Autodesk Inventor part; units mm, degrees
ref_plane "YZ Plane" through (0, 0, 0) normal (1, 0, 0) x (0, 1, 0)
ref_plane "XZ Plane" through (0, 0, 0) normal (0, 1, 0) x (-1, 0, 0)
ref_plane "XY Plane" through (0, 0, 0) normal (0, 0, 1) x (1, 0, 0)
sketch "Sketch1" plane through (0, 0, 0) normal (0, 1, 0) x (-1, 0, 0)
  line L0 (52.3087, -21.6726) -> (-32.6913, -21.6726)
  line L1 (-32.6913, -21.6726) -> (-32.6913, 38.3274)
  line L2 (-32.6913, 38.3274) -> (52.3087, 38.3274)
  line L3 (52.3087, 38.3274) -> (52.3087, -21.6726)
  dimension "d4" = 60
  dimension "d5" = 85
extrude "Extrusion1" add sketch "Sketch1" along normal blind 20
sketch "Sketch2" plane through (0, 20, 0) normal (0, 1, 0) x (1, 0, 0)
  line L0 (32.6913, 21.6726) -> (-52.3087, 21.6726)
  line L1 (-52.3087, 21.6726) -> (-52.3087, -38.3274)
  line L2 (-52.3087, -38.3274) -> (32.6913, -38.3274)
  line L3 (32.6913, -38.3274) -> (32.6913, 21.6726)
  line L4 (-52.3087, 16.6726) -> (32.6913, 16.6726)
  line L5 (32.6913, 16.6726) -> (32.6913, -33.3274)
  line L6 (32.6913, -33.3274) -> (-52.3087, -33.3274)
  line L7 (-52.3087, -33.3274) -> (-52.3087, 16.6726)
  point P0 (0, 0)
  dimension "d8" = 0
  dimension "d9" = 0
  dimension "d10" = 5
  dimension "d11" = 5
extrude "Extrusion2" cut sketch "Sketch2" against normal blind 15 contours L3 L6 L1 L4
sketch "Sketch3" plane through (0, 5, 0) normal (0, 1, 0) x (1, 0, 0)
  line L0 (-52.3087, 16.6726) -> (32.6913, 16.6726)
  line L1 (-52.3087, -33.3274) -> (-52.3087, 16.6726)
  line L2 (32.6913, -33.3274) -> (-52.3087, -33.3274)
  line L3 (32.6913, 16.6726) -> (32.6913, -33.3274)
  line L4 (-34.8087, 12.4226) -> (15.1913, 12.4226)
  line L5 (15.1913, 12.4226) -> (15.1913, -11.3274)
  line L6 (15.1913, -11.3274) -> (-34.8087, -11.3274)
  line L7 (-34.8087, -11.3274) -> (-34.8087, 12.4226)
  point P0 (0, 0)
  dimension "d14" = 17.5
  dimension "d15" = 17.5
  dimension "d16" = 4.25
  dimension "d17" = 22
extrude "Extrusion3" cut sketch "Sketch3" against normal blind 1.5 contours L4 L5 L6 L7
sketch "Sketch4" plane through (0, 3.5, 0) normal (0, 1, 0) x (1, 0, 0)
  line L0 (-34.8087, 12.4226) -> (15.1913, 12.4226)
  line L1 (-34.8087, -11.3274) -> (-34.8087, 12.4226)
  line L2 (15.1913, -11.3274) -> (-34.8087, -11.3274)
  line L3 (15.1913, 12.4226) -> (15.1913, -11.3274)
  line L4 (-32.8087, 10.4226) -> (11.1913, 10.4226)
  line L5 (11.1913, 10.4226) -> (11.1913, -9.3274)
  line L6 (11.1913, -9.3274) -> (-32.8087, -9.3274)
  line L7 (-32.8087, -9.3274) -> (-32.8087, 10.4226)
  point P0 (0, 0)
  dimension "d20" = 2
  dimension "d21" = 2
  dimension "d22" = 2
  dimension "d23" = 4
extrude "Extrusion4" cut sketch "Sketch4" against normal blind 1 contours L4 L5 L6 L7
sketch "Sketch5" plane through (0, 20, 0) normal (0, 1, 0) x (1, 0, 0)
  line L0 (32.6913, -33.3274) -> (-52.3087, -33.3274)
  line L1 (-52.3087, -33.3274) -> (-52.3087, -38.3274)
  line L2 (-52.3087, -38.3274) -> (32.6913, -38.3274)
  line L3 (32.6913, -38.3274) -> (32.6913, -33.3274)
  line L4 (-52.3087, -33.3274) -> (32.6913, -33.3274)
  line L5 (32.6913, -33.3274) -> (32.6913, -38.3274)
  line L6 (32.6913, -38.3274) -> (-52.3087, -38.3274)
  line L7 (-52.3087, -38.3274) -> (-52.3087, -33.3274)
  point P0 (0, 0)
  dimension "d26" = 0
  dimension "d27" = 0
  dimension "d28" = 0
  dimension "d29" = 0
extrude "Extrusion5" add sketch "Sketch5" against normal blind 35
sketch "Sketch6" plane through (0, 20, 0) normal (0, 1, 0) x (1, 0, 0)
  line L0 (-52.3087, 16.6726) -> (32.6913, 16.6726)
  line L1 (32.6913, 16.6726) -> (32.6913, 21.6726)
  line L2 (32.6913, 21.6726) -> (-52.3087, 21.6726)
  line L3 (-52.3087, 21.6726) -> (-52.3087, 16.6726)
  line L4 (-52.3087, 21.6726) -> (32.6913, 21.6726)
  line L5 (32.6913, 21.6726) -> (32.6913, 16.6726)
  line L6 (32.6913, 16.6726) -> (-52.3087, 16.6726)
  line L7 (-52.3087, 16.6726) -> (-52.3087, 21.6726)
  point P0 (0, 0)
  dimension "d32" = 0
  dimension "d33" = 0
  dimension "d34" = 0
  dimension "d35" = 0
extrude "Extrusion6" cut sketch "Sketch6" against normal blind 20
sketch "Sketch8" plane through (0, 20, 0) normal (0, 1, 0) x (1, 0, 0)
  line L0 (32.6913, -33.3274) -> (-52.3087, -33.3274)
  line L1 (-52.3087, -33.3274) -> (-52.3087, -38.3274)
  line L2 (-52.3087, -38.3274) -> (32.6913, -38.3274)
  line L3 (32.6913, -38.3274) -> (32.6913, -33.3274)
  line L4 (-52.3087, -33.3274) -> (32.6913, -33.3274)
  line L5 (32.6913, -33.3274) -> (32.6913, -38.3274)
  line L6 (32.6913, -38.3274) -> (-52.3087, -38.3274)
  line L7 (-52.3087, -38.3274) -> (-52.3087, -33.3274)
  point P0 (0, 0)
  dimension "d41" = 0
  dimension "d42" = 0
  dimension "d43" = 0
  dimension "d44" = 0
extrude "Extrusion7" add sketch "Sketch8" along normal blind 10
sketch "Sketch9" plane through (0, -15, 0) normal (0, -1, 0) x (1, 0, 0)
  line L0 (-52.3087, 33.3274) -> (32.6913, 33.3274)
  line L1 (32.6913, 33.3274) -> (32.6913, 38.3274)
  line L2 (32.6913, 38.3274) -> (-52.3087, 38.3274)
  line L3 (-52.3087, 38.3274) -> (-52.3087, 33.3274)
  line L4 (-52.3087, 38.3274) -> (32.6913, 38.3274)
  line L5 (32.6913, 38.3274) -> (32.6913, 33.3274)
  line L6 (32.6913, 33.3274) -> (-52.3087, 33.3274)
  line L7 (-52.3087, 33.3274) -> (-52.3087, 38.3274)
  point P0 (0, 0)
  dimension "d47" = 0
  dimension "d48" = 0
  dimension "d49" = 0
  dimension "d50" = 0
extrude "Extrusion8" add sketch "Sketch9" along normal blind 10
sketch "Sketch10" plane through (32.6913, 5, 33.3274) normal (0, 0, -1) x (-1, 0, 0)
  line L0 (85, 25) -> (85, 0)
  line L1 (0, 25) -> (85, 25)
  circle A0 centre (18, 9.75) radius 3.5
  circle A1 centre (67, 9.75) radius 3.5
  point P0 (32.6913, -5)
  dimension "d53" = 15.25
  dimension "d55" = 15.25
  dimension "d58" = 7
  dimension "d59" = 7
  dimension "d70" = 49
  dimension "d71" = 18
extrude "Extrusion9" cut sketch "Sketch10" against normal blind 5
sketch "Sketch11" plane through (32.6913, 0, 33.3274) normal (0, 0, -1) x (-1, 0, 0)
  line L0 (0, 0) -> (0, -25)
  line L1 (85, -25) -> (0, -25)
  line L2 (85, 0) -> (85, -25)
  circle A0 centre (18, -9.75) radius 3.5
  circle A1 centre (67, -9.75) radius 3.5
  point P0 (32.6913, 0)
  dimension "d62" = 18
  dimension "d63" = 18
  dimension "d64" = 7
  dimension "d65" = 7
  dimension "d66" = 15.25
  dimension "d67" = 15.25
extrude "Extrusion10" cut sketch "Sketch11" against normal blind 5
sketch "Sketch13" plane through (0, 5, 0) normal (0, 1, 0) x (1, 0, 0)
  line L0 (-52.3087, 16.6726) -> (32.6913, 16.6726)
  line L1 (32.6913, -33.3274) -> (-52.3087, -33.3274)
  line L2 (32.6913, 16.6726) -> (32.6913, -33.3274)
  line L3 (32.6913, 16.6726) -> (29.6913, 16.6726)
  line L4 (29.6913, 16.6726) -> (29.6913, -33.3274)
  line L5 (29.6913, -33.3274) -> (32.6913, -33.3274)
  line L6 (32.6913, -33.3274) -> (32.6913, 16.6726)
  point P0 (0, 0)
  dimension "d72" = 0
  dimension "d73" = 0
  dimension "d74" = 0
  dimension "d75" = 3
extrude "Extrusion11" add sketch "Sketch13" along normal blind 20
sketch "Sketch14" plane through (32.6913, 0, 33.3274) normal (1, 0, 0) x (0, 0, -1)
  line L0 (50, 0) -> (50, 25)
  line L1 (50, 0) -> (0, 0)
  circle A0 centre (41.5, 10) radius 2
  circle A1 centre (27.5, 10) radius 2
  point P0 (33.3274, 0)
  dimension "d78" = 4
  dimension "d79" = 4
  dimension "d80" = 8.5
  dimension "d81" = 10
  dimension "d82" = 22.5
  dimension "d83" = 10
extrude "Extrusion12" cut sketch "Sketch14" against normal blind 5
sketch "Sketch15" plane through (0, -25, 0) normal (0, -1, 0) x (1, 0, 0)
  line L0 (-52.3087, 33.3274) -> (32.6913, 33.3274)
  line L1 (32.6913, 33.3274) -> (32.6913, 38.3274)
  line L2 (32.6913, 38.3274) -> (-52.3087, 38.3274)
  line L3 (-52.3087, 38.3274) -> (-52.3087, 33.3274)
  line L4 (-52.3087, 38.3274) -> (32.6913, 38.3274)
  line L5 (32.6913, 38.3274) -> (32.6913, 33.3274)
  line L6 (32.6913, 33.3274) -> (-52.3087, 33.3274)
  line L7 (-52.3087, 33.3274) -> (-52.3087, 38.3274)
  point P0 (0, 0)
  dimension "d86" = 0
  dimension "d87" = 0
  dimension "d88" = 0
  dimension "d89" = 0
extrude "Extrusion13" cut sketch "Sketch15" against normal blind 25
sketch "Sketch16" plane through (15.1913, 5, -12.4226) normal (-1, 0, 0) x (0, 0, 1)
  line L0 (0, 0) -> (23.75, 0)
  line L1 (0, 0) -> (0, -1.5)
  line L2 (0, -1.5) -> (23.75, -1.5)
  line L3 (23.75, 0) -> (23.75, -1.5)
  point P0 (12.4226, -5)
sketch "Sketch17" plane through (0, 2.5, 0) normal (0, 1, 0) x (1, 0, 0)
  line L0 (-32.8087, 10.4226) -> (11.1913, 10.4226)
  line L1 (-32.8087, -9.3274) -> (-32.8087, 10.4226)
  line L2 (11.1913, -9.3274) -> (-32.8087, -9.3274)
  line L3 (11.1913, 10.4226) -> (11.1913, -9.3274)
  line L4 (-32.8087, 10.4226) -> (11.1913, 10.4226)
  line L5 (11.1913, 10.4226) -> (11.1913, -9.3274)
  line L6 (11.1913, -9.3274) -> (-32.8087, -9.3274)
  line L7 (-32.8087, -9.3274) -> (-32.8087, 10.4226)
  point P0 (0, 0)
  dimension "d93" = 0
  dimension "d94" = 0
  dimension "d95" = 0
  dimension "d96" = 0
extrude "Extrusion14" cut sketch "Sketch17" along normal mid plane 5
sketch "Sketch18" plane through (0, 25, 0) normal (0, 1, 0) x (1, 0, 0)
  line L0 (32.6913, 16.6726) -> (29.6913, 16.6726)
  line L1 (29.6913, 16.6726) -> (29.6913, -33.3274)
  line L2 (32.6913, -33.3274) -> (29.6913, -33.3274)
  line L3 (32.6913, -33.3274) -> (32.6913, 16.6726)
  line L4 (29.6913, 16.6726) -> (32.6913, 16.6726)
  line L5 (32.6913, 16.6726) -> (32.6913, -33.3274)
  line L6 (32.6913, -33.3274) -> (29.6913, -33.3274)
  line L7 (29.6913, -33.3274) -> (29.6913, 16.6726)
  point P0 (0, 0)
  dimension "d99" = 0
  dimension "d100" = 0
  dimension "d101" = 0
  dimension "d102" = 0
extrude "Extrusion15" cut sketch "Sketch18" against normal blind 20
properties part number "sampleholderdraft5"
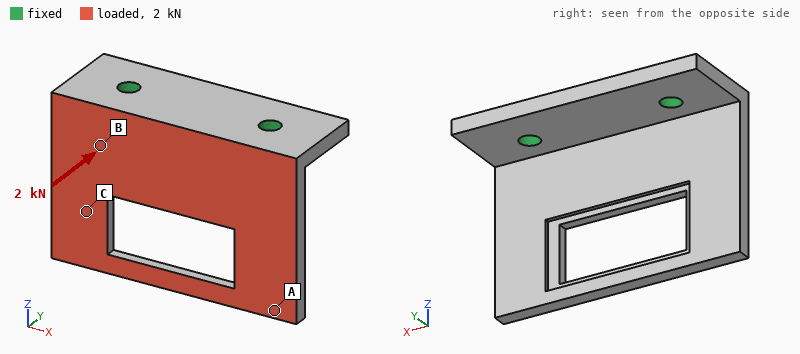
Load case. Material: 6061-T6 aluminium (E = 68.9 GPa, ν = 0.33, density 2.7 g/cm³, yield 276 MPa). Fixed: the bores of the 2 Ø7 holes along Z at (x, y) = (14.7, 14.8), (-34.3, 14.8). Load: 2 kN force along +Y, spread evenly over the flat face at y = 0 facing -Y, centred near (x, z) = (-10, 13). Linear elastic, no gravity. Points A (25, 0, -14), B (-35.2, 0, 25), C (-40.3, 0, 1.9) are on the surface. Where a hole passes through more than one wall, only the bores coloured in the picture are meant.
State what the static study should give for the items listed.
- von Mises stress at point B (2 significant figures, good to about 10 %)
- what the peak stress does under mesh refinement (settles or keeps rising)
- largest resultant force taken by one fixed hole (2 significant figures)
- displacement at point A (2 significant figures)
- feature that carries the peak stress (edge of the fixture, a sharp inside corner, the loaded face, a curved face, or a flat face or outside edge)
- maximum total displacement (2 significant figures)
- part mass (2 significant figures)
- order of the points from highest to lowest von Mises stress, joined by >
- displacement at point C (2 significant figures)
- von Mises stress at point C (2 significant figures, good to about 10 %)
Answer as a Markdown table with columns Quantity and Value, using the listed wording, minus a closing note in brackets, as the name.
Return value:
| Quantity | Value |
|---|---|
| von Mises stress at point B | 77 MPa |
| what the peak stress does under mesh refinement | keeps rising |
| largest resultant force taken by one fixed hole | 1.0 kN |
| displacement at point A | 0.96 mm |
| feature that carries the peak stress | edge of the fixture |
| maximum total displacement | 1.0 mm |
| part mass | 78 g |
| order of the points from highest to lowest von Mises stress, joined by > | B > C > A |
| displacement at point C | 0.57 mm |
| von Mises stress at point C | 44 MPa |
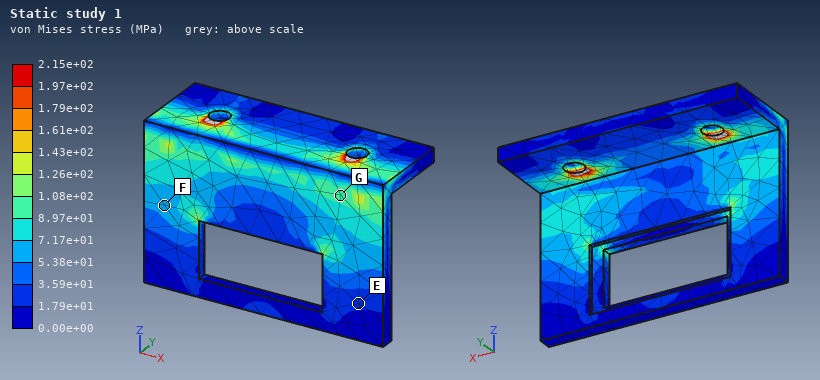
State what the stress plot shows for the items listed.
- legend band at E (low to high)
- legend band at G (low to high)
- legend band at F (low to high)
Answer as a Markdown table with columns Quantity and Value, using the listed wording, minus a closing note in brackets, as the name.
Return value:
| Quantity | Value |
|---|---|
| legend band at E | 1.79e+01 to 3.59e+01 MPa |
| legend band at G | 8.97e+01 to 1.08e+02 MPa |
| legend band at F | 5.38e+01 to 7.17e+01 MPa |
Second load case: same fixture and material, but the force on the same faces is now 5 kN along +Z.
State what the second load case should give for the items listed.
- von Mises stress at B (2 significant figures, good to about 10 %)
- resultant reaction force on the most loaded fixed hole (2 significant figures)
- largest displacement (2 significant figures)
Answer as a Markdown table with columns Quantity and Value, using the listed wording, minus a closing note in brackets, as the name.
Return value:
| Quantity | Value |
|---|---|
| von Mises stress at B | 41 MPa |
| resultant reaction force on the most loaded fixed hole | 2.5 kN |
| largest displacement | 0.66 mm |
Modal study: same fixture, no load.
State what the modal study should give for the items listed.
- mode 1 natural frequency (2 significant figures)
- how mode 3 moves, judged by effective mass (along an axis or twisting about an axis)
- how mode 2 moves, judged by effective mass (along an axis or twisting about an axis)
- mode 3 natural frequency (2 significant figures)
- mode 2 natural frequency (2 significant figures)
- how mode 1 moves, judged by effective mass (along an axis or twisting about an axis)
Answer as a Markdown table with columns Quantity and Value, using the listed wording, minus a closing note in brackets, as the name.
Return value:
| Quantity | Value |
|---|---|
| mode 1 natural frequency | 1200 Hz |
| how mode 3 moves, judged by effective mass | along X |
| how mode 2 moves, judged by effective mass | twisting about Z |
| mode 3 natural frequency | 4500 Hz |
| mode 2 natural frequency | 1900 Hz |
| how mode 1 moves, judged by effective mass | along Y |
